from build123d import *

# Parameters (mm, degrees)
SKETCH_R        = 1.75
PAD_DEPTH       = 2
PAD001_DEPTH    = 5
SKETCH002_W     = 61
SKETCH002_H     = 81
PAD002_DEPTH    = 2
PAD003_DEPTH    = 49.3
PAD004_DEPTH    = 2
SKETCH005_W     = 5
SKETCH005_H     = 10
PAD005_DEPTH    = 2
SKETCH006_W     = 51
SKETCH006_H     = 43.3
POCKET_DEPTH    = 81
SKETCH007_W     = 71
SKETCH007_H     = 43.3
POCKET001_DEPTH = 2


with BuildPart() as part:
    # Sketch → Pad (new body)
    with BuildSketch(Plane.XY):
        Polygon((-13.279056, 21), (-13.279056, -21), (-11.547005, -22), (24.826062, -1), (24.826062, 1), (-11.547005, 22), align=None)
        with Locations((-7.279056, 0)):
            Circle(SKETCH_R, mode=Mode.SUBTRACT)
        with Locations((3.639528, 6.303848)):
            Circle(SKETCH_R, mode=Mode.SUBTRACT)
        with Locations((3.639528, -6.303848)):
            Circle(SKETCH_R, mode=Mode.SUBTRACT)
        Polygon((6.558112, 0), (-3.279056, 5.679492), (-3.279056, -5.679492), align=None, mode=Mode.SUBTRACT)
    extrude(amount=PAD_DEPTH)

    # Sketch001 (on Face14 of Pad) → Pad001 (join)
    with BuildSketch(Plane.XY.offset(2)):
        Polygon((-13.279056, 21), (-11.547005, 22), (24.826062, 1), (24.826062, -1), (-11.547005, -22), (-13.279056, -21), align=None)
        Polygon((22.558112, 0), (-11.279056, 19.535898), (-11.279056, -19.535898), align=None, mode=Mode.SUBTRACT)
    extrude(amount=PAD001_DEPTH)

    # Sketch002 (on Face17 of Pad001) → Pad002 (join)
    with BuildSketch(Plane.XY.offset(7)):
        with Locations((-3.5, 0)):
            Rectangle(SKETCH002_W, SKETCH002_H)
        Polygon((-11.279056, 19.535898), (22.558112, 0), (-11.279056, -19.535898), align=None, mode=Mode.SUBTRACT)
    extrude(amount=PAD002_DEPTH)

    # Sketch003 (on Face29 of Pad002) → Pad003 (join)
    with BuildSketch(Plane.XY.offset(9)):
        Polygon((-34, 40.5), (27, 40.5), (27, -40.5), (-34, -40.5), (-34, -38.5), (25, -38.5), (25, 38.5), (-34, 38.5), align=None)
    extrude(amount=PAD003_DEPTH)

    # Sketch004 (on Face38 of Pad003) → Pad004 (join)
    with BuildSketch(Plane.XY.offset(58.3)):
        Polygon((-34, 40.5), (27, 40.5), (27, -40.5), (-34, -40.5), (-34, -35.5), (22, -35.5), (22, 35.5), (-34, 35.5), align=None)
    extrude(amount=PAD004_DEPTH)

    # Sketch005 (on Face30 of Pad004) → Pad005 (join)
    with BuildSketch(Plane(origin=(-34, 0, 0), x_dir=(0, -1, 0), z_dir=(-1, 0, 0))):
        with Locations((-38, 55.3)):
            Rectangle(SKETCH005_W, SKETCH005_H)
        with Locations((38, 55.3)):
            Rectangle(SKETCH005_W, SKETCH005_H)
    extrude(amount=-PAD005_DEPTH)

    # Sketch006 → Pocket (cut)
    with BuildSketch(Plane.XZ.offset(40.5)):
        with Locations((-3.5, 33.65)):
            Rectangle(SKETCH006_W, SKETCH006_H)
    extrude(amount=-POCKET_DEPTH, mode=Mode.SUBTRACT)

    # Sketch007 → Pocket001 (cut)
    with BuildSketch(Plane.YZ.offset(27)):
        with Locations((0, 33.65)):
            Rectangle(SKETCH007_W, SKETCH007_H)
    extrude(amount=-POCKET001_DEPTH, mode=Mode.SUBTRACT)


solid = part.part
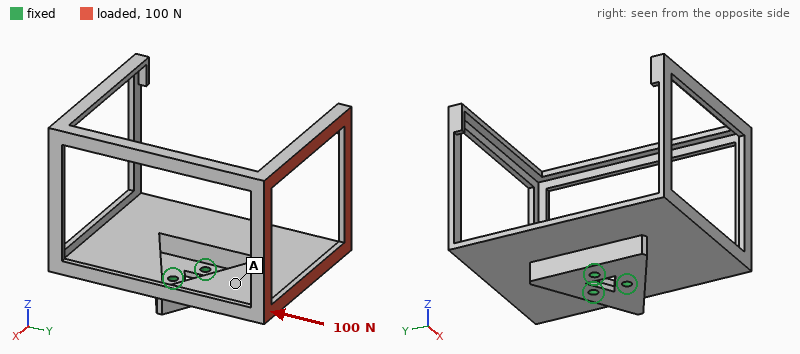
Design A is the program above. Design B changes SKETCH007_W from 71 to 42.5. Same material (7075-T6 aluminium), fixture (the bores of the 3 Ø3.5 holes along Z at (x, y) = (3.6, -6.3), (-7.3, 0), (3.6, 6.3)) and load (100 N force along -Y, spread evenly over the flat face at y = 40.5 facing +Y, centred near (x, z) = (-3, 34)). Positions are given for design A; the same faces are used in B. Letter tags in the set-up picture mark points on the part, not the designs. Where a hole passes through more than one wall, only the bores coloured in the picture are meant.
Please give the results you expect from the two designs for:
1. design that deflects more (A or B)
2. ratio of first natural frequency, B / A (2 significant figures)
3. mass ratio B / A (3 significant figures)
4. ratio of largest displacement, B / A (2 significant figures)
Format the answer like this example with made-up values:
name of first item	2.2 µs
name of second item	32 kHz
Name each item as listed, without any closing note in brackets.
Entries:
design that deflects more	A
ratio of first natural frequency, B / A	1.0
mass ratio B / A	1.14
ratio of largest displacement, B / A	0.85
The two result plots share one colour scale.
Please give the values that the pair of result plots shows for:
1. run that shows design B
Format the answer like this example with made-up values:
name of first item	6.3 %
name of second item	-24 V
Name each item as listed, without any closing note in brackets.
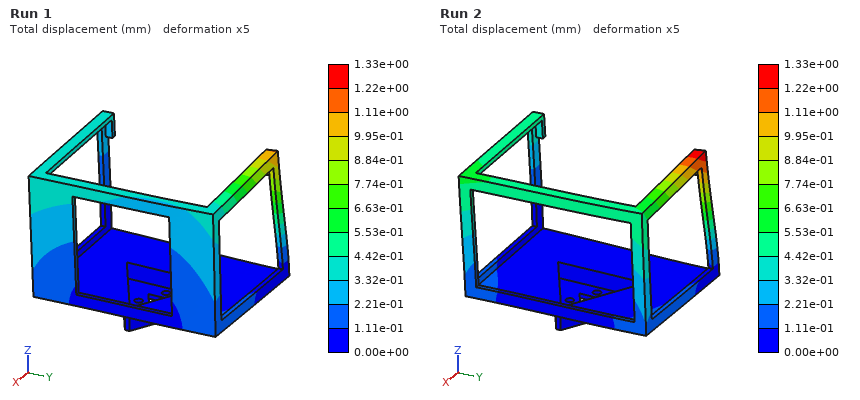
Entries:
run that shows design B	Run 1
